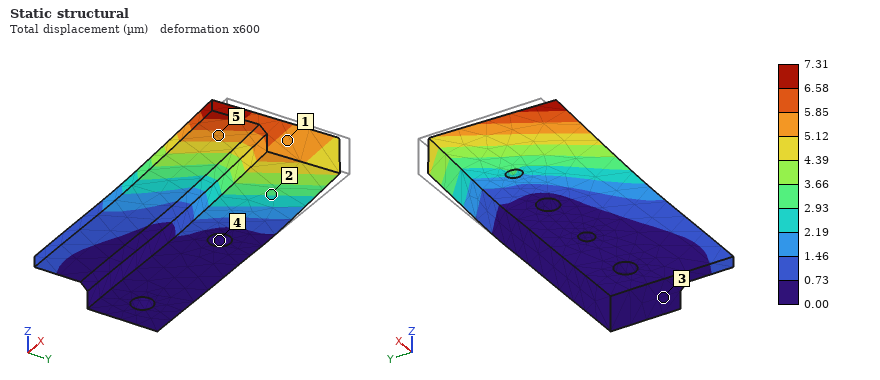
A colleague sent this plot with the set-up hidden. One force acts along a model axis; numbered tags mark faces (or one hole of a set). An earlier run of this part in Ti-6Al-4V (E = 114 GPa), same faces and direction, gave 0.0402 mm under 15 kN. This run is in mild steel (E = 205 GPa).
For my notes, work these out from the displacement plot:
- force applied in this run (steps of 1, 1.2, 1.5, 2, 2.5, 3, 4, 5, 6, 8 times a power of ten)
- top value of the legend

5 kN
7.31 µm
